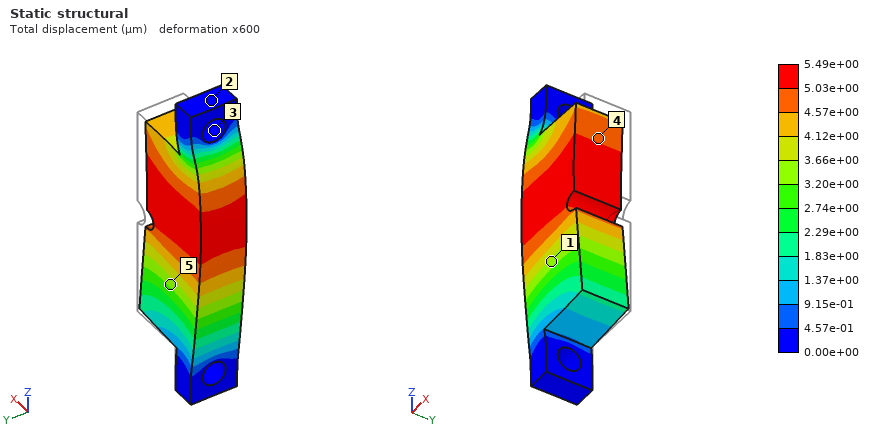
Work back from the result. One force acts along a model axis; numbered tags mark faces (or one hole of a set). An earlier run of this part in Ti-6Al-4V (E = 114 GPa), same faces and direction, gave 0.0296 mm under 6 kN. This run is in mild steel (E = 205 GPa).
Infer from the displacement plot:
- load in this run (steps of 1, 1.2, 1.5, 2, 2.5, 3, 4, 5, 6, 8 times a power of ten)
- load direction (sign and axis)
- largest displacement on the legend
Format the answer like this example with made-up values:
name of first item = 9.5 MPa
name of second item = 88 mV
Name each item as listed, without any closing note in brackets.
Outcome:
load in this run = 2 kN
load direction = -X
largest displacement on the legend = 5.49e+00 µm
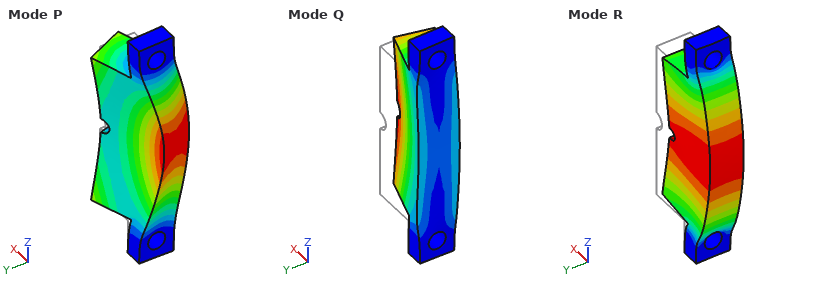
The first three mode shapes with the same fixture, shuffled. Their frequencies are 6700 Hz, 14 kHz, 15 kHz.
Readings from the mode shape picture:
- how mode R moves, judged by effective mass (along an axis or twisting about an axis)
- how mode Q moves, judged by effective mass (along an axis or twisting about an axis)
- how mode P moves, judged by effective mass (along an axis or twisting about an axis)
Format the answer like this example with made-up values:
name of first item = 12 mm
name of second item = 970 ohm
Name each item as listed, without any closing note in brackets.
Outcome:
how mode R moves, judged by effective mass = along X
how mode Q moves, judged by effective mass = along Y
how mode P moves, judged by effective mass = along Y
